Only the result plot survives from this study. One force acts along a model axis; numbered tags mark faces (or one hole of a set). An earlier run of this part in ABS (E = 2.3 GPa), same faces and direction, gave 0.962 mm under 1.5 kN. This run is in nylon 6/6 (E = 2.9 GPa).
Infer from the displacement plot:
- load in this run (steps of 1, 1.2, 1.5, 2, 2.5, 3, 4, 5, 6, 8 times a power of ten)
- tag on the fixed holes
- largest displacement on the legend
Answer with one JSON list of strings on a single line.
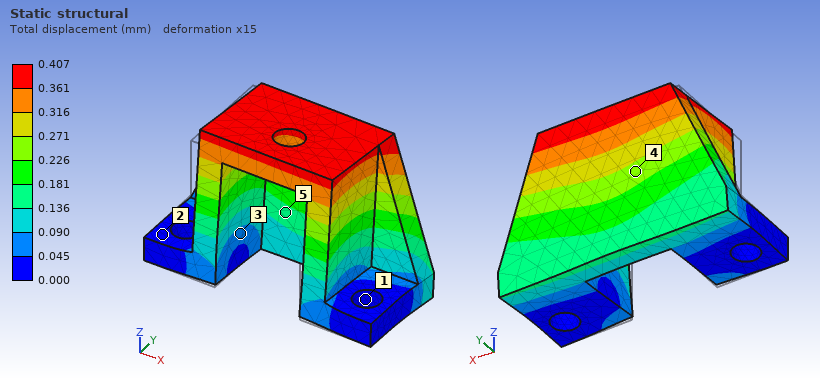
["800 N", "1", "0.407 mm"]
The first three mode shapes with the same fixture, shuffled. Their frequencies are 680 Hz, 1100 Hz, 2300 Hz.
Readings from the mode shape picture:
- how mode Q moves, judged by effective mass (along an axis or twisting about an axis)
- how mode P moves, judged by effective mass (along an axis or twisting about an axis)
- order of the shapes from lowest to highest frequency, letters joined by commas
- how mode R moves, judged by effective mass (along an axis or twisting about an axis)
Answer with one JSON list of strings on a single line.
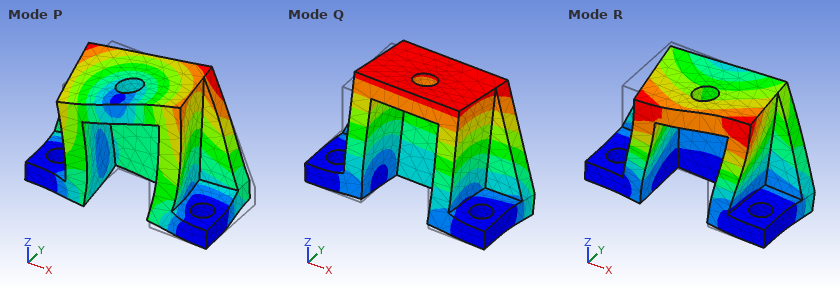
["along Y", "along X", "Q, R, P", "along X"]
